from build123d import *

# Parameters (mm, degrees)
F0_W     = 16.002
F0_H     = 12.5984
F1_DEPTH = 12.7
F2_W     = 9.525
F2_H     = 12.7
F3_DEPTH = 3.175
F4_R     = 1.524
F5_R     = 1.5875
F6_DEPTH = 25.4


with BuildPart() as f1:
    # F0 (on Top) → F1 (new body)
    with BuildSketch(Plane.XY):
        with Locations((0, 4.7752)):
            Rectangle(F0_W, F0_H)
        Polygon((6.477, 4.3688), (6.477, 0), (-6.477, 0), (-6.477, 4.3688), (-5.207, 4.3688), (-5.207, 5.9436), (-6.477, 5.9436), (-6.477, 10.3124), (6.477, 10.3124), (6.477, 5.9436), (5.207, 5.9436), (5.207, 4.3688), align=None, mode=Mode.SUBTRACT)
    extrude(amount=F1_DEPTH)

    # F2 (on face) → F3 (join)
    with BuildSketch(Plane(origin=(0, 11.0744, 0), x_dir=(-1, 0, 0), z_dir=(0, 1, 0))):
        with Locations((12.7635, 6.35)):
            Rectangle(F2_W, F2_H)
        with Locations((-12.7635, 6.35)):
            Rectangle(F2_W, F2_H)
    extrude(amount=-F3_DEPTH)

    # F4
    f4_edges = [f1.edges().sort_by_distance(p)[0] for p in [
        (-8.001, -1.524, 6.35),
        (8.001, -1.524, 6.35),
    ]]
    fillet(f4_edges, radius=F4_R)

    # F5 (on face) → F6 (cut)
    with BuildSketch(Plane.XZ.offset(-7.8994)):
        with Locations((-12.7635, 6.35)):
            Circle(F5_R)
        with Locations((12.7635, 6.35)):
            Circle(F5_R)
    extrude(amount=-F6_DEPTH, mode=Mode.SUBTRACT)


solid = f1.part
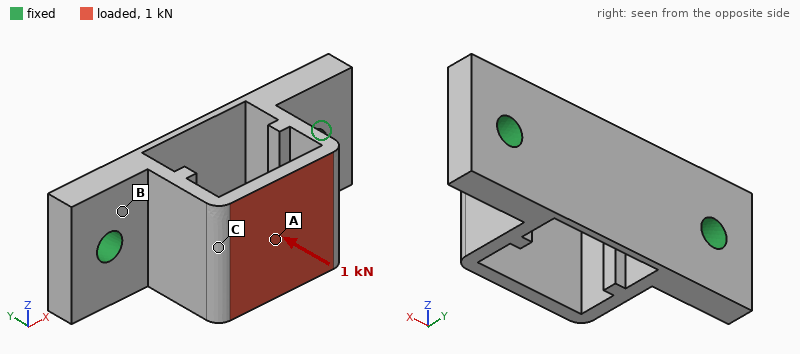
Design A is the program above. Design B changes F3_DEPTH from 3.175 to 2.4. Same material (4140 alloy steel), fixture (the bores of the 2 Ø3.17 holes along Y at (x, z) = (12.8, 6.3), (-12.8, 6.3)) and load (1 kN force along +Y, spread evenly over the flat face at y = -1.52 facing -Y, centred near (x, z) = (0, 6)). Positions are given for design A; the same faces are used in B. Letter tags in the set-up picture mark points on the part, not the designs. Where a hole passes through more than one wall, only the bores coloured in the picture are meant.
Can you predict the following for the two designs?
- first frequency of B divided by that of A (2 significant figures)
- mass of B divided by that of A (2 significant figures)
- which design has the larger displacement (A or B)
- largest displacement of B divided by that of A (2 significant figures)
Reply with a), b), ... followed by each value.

a) 0.86
b) 0.89
c) B
d) 1.1
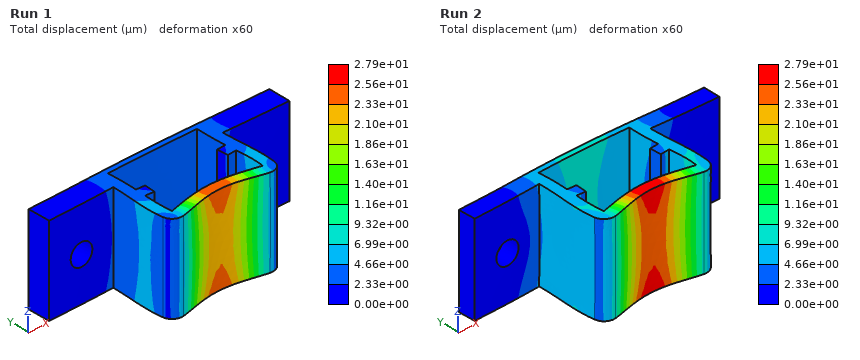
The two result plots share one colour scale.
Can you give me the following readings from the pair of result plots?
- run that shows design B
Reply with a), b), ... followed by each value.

a) Run 2
